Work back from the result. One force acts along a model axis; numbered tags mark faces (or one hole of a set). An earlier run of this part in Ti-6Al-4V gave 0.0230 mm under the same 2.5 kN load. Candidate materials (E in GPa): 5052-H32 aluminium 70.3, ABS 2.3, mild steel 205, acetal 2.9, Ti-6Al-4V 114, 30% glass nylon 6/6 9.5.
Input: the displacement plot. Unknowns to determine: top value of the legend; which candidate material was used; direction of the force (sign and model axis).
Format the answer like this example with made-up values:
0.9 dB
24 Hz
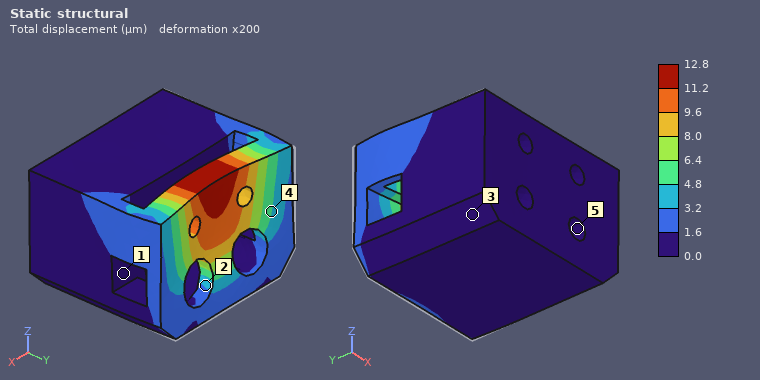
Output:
12.8 µm
mild steel
-Y
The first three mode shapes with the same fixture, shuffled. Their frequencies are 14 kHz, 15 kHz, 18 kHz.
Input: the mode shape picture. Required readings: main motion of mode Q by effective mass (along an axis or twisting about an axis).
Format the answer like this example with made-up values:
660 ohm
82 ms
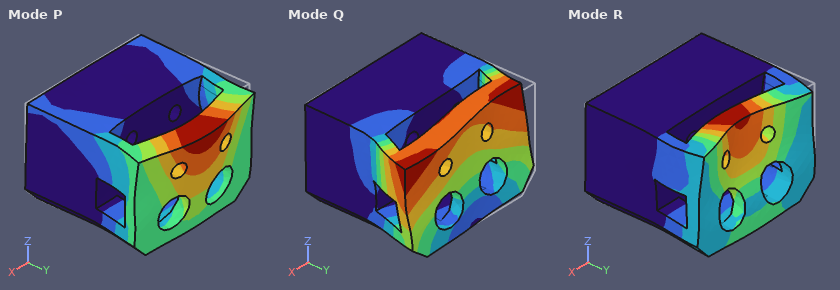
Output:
along X
